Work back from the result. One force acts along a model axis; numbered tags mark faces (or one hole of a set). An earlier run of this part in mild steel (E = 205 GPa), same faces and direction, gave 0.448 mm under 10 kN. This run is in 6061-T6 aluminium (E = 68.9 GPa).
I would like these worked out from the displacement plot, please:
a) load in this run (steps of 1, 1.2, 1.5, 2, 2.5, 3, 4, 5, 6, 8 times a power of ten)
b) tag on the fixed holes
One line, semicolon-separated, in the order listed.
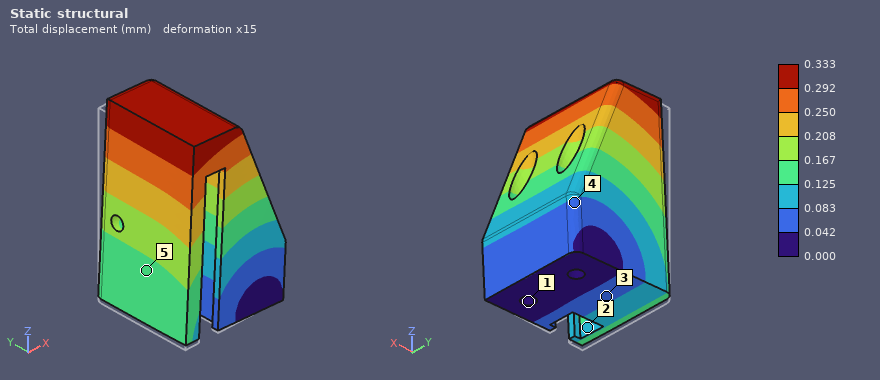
2.5 kN; 1
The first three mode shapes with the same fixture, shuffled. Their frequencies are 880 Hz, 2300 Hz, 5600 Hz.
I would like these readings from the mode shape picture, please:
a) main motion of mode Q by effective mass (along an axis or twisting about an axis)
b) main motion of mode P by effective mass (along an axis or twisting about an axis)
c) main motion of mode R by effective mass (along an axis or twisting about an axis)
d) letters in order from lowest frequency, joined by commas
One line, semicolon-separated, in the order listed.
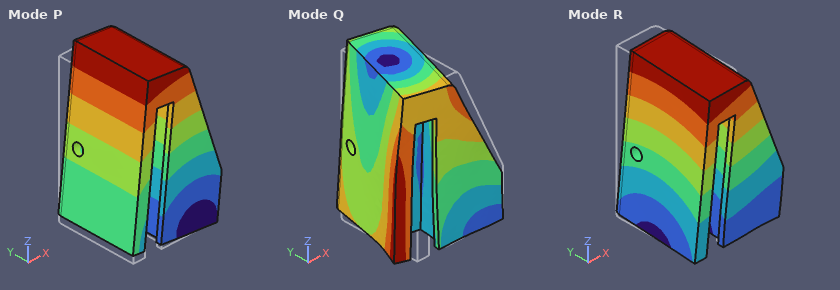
twisting about Z; along X; along Y; P, R, Q
